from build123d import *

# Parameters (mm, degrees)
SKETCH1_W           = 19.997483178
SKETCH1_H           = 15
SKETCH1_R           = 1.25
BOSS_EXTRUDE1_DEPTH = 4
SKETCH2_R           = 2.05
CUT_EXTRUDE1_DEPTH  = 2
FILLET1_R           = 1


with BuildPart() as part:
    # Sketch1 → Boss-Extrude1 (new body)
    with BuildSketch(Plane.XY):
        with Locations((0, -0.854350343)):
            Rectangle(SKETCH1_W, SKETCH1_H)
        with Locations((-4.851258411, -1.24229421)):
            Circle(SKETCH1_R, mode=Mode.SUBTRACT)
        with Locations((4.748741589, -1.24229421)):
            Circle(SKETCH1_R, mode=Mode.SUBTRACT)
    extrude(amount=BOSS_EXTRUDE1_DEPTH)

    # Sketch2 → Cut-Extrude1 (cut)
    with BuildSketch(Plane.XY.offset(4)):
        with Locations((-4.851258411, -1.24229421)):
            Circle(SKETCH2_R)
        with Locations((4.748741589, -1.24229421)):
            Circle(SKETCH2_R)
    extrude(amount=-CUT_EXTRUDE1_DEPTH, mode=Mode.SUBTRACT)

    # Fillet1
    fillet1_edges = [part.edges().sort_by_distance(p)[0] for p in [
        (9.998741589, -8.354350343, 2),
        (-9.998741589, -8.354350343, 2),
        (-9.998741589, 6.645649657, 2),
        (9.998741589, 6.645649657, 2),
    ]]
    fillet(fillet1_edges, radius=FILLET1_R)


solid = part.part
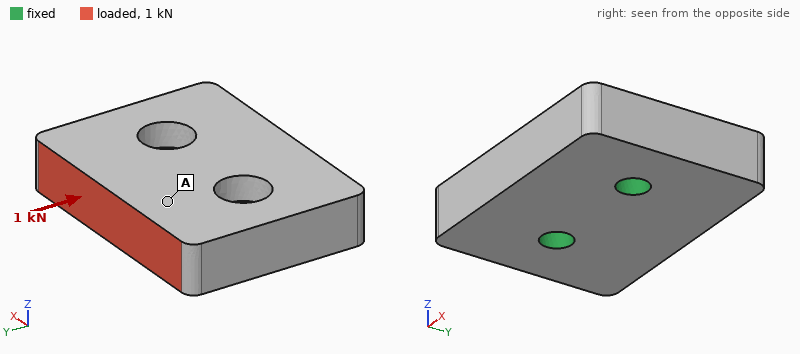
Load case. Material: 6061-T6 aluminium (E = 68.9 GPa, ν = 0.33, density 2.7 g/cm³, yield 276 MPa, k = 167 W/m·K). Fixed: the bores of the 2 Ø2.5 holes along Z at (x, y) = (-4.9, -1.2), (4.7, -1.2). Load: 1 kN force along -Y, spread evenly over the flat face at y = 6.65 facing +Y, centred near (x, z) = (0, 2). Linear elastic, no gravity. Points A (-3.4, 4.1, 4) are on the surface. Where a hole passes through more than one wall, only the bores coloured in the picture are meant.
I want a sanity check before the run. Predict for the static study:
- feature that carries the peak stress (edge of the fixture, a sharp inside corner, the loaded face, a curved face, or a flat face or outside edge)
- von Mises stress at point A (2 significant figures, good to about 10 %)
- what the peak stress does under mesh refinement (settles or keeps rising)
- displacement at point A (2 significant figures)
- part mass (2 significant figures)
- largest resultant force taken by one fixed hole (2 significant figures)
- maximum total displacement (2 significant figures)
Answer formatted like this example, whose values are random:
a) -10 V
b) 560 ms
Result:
a) edge of the fixture
b) 13 MPa
c) keeps rising
d) 6.6 µm
e) 3.0 g
f) 510 N
g) 8.9 µm
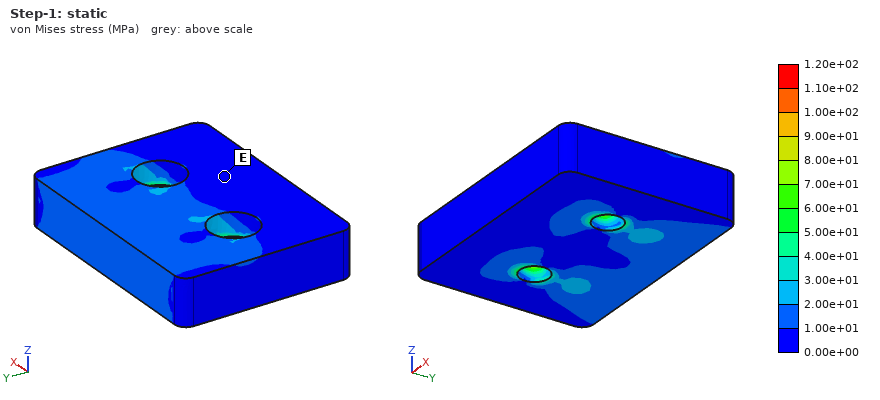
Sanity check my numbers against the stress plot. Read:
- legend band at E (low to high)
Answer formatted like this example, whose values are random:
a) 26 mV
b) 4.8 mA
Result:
a) 0.00e+00 to 1.00e+01 MPa
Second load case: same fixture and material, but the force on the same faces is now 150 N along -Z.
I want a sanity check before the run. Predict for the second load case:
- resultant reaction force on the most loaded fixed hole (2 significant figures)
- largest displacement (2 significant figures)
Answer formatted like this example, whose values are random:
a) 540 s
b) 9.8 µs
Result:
a) 76 N
b) 11 µm
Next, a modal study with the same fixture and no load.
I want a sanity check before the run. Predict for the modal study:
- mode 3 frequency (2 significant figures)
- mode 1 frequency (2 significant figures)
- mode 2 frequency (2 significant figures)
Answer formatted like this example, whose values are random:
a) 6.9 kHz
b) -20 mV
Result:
a) 44 kHz
b) 22 kHz
c) 38 kHz
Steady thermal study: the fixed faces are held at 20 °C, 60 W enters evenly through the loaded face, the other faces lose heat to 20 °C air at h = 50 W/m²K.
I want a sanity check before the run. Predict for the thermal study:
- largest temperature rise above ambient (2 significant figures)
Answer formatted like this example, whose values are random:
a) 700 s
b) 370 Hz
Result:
a) 46 K
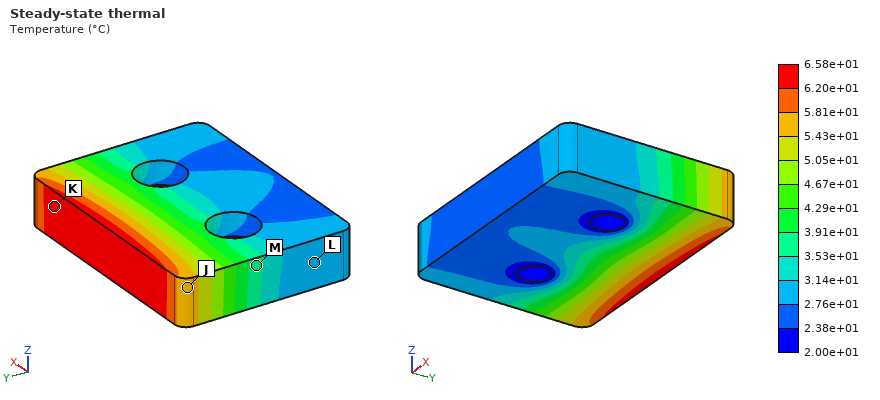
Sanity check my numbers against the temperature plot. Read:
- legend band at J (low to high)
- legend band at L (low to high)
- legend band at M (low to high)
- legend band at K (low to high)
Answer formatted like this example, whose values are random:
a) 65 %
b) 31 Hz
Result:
a) 5.43e+01 to 5.81e+01 °C
b) 2.76e+01 to 3.14e+01 °C
c) 3.53e+01 to 3.91e+01 °C
d) 6.20e+01 to 6.58e+01 °C
